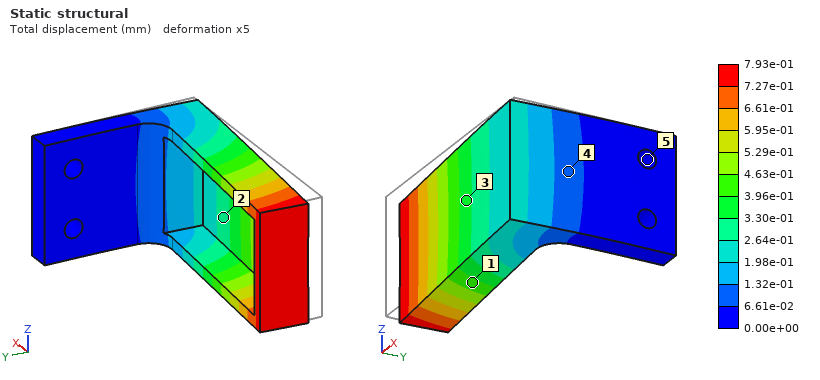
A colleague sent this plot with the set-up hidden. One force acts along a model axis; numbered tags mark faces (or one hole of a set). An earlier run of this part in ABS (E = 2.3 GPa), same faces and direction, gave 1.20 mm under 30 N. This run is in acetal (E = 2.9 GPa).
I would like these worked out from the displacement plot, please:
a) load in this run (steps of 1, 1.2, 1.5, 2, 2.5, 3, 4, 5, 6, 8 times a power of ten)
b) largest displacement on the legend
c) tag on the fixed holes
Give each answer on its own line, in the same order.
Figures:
25 N
7.93e-01 mm
5
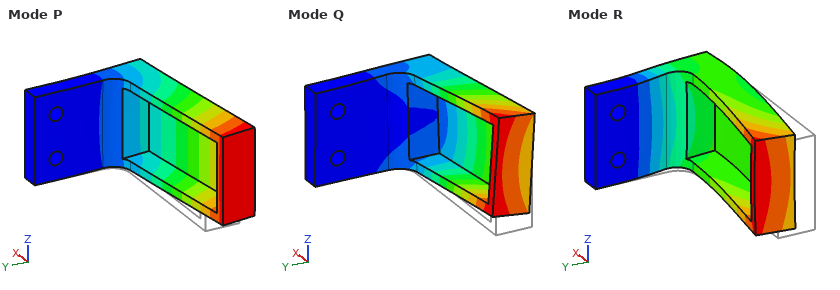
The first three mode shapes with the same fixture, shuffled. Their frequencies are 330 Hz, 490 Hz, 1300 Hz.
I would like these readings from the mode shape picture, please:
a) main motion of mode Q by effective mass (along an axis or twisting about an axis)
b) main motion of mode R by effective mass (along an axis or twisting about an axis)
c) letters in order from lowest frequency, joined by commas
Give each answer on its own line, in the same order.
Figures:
along Z
along X
P, Q, R
